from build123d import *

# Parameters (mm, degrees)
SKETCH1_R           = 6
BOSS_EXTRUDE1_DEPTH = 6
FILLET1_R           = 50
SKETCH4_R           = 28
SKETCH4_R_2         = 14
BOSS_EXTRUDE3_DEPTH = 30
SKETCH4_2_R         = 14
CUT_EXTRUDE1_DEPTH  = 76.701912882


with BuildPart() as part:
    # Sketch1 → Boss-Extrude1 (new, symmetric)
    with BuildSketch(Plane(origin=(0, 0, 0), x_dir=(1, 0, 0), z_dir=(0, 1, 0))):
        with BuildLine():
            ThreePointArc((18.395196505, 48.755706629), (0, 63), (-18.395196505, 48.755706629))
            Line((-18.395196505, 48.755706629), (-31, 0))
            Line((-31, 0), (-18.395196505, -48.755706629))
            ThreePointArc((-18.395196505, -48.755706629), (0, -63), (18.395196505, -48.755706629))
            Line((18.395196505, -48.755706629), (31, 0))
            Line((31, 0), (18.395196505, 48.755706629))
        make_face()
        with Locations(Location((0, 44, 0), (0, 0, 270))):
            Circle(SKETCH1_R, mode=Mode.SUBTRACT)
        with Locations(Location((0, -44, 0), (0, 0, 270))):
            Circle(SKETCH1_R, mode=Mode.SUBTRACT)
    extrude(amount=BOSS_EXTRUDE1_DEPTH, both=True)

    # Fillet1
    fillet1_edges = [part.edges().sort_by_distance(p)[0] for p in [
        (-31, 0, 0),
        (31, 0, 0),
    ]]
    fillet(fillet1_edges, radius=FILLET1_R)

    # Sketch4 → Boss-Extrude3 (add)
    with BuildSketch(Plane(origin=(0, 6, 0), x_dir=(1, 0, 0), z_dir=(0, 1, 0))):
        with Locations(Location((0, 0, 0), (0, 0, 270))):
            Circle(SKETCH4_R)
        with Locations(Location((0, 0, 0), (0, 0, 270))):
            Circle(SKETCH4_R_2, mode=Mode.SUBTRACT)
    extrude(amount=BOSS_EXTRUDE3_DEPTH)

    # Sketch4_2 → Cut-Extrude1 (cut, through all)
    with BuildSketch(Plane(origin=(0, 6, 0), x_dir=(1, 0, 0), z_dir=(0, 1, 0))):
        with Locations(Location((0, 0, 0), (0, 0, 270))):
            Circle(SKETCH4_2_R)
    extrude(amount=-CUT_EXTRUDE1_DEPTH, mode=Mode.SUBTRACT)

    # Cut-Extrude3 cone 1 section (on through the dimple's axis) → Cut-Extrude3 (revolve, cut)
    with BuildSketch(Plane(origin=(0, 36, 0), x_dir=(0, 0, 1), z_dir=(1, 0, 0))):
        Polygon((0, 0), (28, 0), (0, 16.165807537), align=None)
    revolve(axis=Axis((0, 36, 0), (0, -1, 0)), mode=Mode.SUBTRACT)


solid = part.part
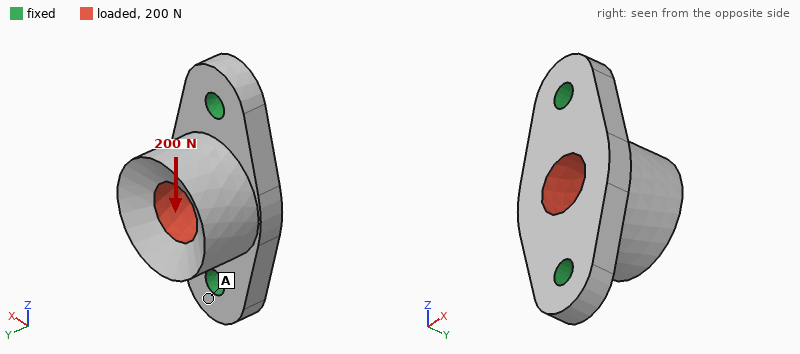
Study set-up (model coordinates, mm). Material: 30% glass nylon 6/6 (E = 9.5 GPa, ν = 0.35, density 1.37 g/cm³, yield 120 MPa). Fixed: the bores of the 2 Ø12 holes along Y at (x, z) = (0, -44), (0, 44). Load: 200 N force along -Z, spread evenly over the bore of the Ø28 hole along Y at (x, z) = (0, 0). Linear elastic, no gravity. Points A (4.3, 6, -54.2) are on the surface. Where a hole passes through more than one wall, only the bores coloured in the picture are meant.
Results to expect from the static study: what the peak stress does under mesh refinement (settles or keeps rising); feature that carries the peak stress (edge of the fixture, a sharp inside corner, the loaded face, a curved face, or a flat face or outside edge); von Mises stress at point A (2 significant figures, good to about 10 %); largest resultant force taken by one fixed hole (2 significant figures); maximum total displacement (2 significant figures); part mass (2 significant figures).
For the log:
keeps rising
edge of the fixture
0.050 MPa
100 N
1.8 µm
140 g
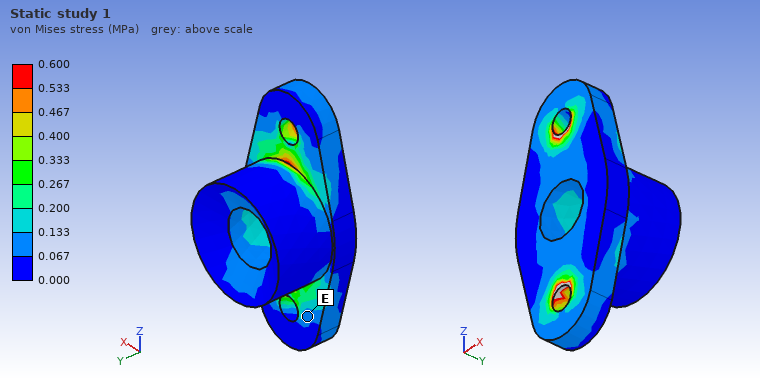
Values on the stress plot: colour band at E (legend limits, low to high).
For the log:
0.067 to 0.133 MPa
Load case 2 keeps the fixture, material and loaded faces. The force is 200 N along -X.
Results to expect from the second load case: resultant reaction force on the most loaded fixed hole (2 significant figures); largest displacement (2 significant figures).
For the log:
100 N
13 µm
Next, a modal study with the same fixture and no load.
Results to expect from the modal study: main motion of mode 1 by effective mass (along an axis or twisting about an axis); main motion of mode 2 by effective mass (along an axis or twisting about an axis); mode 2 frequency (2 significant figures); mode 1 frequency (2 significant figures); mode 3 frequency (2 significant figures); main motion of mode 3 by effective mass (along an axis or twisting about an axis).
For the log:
along X
along Y
3600 Hz
2000 Hz
5300 Hz
along Z
